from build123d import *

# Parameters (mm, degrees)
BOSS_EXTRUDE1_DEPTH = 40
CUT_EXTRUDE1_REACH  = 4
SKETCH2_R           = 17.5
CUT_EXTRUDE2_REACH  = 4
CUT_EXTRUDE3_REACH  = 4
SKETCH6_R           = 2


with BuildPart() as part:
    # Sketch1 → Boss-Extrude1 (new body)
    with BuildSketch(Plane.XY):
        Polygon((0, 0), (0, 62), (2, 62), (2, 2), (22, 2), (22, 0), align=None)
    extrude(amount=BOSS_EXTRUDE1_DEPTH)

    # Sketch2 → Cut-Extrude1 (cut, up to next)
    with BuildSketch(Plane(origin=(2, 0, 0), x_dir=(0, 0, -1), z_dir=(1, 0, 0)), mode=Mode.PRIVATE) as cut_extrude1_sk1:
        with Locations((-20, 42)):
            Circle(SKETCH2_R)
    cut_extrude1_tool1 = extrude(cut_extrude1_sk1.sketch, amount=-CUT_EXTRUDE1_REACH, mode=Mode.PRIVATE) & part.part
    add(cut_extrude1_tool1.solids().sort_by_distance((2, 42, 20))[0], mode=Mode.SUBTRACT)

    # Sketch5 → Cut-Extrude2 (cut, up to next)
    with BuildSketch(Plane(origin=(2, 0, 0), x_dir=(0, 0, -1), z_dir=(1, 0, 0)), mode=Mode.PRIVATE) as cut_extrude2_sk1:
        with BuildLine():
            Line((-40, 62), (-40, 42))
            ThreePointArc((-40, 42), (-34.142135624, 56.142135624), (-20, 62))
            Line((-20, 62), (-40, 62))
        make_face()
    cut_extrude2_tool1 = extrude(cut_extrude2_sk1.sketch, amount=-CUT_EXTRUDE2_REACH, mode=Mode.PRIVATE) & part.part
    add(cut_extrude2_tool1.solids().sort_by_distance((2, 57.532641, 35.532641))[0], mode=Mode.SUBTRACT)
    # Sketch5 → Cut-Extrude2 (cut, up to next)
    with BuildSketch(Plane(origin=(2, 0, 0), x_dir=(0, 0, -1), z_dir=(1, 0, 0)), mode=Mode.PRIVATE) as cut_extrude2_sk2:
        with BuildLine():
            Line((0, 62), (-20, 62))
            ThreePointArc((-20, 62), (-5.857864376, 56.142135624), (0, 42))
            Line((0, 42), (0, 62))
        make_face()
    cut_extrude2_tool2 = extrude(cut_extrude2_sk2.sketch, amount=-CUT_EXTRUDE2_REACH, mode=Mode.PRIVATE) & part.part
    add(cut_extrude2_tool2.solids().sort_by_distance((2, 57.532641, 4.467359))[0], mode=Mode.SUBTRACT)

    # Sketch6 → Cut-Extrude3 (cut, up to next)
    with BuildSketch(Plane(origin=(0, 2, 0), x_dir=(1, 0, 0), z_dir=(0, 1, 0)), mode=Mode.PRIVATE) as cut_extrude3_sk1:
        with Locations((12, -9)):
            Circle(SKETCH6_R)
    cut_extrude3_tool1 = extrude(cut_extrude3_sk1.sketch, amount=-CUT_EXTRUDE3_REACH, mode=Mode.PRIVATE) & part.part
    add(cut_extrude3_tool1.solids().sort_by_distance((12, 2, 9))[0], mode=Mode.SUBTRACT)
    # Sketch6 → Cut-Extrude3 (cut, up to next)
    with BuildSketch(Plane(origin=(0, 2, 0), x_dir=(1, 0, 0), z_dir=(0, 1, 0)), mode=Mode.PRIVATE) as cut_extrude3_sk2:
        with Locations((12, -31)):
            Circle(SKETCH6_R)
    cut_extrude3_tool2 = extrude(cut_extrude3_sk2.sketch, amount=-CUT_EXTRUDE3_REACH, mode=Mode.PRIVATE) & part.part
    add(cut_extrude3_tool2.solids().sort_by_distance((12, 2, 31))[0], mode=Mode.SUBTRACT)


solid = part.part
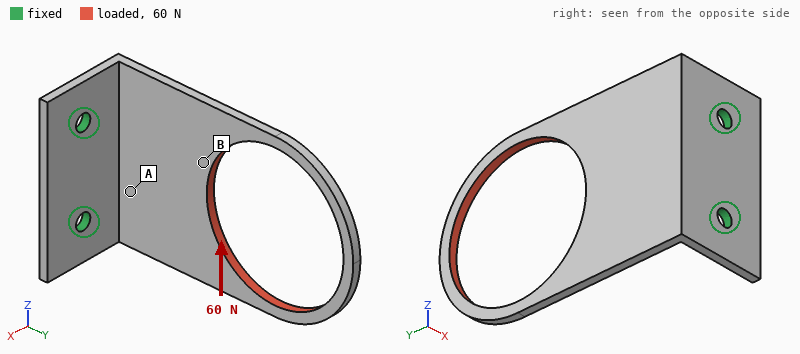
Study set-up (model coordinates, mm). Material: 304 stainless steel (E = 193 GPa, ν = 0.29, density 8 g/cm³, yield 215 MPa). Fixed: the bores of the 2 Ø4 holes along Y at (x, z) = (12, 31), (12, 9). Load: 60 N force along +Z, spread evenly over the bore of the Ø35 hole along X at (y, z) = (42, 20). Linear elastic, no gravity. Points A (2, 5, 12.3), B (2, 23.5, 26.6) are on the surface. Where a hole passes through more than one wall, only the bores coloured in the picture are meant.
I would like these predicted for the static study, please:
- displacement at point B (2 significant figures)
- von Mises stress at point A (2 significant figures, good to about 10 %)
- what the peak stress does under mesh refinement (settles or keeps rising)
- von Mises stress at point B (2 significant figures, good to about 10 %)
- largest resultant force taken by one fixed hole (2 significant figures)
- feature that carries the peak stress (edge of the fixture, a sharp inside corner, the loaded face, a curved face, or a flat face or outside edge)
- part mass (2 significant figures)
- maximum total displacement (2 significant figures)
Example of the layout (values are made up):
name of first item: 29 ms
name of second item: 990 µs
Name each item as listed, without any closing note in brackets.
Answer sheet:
displacement at point B: 19 µm
von Mises stress at point A: 18 MPa
what the peak stress does under mesh refinement: keeps rising
von Mises stress at point B: 7.1 MPa
largest resultant force taken by one fixed hole: 100 N
feature that carries the peak stress: edge of the fixture
part mass: 34 g
maximum total displacement: 70 µm
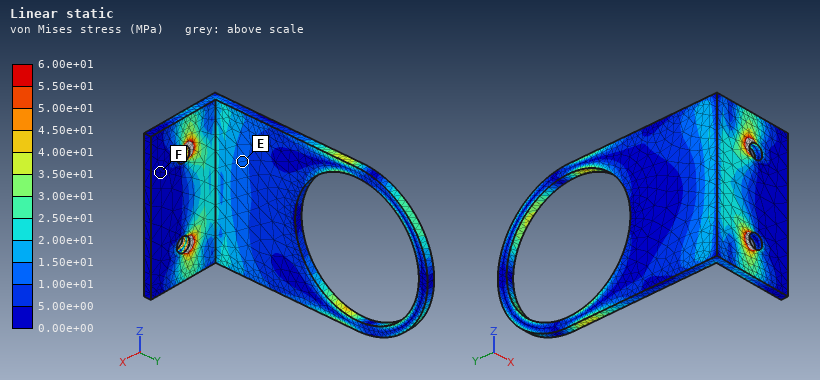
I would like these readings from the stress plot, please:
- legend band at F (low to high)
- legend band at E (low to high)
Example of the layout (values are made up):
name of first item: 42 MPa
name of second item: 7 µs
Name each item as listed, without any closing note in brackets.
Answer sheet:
legend band at F: 0.00e+00 to 5.00e+00 MPa
legend band at E: 1.00e+01 to 1.50e+01 MPa
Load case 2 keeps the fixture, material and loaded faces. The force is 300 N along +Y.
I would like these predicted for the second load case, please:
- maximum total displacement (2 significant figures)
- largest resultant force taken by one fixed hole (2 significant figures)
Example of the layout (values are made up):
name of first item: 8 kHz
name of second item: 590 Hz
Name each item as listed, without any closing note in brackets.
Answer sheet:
maximum total displacement: 0.20 mm
largest resultant force taken by one fixed hole: 150 N
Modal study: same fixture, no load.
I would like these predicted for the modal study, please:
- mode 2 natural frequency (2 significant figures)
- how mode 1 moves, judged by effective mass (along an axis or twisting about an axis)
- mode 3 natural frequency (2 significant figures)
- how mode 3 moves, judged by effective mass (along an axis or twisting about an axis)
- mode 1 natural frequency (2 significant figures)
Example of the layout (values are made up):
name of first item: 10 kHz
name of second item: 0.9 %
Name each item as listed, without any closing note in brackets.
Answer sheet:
mode 2 natural frequency: 1600 Hz
how mode 1 moves, judged by effective mass: along X
mode 3 natural frequency: 1900 Hz
how mode 3 moves, judged by effective mass: along X
mode 1 natural frequency: 630 Hz
